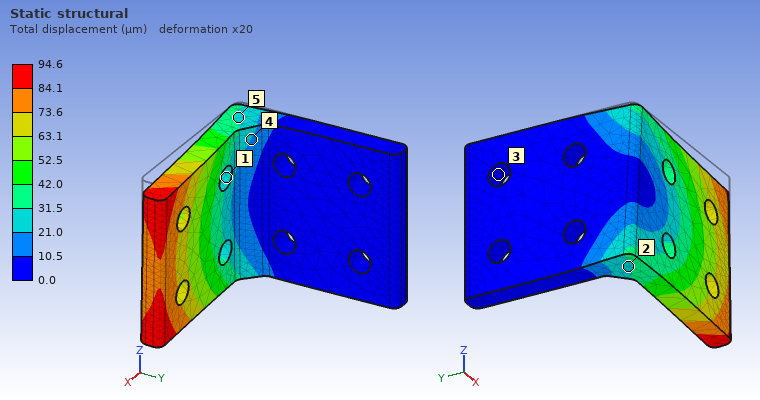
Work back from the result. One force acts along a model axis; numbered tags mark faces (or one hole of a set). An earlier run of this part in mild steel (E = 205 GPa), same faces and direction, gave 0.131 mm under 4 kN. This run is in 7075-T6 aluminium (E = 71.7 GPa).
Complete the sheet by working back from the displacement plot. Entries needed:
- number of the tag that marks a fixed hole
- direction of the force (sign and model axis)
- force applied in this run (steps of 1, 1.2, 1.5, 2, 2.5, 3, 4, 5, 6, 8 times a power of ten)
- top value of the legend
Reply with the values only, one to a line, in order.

3
-Z
1 kN
94.6 µm
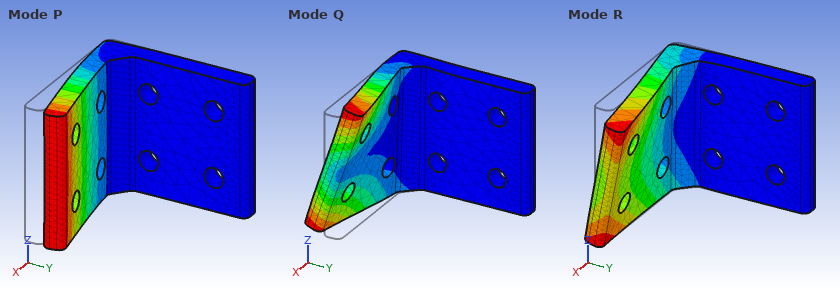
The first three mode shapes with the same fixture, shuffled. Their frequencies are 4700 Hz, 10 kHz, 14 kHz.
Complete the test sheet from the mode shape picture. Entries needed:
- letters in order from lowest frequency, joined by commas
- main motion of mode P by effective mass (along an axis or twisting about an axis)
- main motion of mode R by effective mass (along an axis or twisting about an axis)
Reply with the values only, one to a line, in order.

P, R, Q
along Y
along Z
